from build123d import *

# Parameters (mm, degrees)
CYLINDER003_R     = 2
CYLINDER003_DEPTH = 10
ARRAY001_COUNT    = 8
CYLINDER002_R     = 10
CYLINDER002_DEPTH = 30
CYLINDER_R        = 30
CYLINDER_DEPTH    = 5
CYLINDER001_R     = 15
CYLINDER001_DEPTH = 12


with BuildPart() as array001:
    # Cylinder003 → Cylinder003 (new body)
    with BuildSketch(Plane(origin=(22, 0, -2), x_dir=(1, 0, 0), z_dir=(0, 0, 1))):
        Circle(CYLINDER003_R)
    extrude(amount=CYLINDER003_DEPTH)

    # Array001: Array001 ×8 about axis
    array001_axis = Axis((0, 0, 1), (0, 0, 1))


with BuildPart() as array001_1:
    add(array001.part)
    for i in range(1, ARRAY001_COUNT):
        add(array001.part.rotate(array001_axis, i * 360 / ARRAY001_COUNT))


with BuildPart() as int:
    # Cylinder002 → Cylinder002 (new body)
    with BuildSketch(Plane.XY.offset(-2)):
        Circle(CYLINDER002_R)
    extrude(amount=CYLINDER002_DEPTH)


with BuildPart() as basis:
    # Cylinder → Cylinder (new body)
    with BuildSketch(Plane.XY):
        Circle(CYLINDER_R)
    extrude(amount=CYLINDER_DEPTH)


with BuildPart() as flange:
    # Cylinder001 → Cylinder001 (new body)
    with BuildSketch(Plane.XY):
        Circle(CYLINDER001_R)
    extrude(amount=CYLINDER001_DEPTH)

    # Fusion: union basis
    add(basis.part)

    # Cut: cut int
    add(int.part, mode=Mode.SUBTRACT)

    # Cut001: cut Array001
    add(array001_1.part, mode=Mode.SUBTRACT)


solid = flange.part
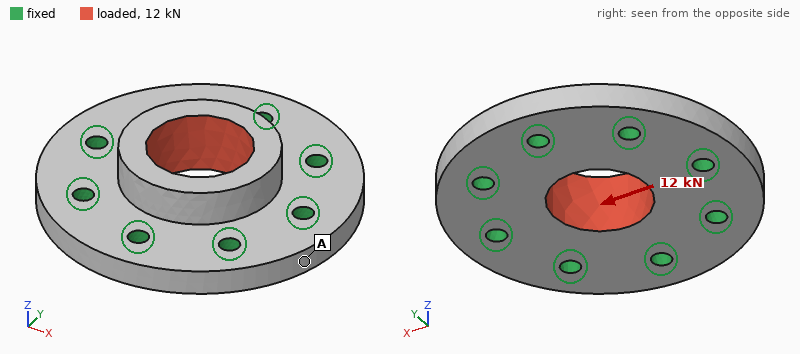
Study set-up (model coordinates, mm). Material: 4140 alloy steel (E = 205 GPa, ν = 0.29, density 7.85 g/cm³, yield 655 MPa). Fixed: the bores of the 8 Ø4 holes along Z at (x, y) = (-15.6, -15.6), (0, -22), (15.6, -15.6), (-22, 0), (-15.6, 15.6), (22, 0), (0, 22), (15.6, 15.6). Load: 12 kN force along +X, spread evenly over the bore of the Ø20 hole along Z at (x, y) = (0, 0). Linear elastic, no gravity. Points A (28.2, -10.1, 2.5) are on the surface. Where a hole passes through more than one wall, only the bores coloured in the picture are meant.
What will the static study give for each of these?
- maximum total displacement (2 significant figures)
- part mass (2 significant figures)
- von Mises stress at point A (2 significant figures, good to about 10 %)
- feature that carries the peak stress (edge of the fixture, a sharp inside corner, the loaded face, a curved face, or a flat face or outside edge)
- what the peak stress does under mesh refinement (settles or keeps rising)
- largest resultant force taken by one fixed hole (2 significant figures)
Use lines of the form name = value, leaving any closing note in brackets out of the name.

maximum total displacement = 5.7 µm
part mass = 120 g
von Mises stress at point A = 9.3 MPa
feature that carries the peak stress = edge of the fixture
what the peak stress does under mesh refinement = keeps rising
largest resultant force taken by one fixed hole = 2.2 kN
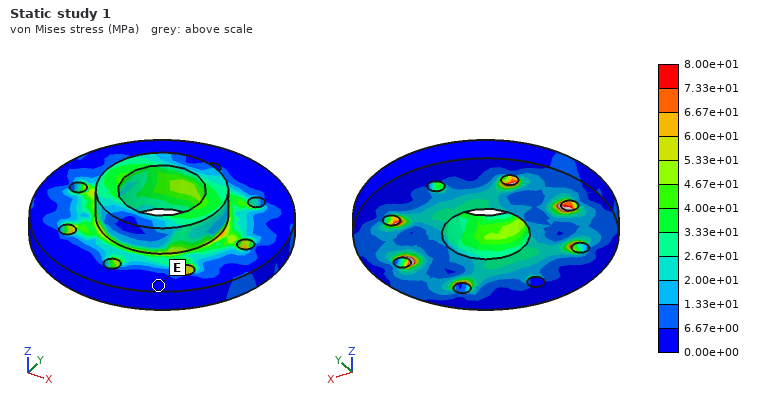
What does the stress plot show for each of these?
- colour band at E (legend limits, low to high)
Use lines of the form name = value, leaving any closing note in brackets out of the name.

colour band at E = 0.00e+00 to 6.67e+00 MPa
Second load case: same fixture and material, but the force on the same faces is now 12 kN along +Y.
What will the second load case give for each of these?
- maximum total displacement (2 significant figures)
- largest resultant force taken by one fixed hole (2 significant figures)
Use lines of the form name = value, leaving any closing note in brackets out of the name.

maximum total displacement = 5.7 µm
largest resultant force taken by one fixed hole = 2.2 kN
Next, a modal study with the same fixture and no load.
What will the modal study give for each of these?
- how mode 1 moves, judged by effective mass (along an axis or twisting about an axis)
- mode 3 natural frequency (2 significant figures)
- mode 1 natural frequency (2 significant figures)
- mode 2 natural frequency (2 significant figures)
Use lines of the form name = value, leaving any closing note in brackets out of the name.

how mode 1 moves, judged by effective mass = along Z
mode 3 natural frequency = 38 kHz
mode 1 natural frequency = 30 kHz
mode 2 natural frequency = 38 kHz
